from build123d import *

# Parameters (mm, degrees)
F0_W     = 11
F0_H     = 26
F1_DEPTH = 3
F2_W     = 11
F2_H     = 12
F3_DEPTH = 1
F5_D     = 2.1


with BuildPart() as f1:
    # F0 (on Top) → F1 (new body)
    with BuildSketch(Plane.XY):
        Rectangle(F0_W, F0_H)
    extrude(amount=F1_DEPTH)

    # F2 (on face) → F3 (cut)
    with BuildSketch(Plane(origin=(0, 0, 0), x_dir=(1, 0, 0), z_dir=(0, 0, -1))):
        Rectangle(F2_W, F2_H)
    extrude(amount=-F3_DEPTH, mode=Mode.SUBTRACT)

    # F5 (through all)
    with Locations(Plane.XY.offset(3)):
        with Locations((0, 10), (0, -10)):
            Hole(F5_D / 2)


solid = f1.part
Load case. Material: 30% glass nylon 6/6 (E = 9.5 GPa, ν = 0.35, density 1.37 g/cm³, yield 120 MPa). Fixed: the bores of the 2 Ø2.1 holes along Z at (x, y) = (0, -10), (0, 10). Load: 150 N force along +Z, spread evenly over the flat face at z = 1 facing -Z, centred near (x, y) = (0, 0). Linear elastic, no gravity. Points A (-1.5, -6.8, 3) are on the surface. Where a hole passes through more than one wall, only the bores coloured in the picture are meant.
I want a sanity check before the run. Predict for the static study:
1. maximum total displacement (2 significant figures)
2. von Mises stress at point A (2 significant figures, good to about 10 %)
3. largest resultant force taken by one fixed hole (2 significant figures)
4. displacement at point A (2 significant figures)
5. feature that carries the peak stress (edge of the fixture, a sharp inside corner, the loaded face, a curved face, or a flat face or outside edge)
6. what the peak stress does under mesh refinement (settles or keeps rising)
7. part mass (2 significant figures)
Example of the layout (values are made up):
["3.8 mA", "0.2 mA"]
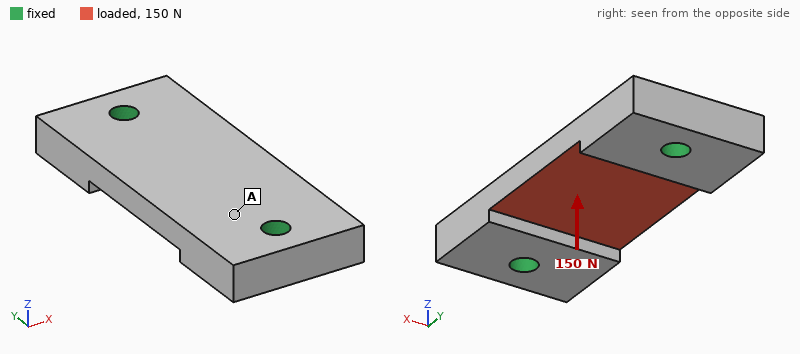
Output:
["48 µm", "11 MPa", "83 N", "12 µm", "edge of the fixture", "keeps rising", "0.97 g"]
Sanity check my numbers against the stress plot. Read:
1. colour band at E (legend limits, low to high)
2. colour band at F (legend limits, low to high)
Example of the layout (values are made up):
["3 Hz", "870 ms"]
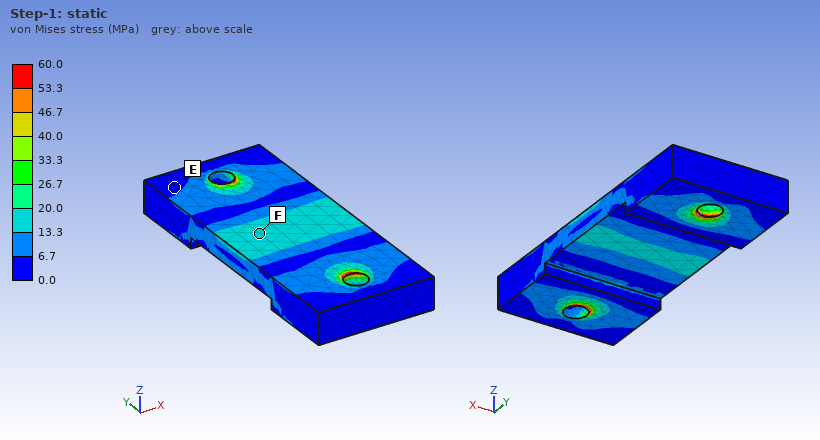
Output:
["0.0 to 6.7 MPa", "13.3 to 20.0 MPa"]
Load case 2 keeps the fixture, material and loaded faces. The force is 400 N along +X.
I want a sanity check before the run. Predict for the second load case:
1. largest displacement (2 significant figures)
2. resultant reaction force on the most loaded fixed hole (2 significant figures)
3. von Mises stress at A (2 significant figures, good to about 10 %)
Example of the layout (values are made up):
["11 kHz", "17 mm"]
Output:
["49 µm", "200 N", "11 MPa"]
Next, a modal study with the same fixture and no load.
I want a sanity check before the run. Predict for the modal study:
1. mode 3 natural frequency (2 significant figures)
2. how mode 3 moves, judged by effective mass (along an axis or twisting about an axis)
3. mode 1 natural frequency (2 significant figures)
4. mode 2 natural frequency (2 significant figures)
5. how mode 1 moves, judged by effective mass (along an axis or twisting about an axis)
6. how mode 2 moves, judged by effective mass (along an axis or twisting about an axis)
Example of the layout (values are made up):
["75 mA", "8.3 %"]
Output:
["28 kHz", "along X", "17 kHz", "19 kHz", "along Z", "twisting about Y"]
